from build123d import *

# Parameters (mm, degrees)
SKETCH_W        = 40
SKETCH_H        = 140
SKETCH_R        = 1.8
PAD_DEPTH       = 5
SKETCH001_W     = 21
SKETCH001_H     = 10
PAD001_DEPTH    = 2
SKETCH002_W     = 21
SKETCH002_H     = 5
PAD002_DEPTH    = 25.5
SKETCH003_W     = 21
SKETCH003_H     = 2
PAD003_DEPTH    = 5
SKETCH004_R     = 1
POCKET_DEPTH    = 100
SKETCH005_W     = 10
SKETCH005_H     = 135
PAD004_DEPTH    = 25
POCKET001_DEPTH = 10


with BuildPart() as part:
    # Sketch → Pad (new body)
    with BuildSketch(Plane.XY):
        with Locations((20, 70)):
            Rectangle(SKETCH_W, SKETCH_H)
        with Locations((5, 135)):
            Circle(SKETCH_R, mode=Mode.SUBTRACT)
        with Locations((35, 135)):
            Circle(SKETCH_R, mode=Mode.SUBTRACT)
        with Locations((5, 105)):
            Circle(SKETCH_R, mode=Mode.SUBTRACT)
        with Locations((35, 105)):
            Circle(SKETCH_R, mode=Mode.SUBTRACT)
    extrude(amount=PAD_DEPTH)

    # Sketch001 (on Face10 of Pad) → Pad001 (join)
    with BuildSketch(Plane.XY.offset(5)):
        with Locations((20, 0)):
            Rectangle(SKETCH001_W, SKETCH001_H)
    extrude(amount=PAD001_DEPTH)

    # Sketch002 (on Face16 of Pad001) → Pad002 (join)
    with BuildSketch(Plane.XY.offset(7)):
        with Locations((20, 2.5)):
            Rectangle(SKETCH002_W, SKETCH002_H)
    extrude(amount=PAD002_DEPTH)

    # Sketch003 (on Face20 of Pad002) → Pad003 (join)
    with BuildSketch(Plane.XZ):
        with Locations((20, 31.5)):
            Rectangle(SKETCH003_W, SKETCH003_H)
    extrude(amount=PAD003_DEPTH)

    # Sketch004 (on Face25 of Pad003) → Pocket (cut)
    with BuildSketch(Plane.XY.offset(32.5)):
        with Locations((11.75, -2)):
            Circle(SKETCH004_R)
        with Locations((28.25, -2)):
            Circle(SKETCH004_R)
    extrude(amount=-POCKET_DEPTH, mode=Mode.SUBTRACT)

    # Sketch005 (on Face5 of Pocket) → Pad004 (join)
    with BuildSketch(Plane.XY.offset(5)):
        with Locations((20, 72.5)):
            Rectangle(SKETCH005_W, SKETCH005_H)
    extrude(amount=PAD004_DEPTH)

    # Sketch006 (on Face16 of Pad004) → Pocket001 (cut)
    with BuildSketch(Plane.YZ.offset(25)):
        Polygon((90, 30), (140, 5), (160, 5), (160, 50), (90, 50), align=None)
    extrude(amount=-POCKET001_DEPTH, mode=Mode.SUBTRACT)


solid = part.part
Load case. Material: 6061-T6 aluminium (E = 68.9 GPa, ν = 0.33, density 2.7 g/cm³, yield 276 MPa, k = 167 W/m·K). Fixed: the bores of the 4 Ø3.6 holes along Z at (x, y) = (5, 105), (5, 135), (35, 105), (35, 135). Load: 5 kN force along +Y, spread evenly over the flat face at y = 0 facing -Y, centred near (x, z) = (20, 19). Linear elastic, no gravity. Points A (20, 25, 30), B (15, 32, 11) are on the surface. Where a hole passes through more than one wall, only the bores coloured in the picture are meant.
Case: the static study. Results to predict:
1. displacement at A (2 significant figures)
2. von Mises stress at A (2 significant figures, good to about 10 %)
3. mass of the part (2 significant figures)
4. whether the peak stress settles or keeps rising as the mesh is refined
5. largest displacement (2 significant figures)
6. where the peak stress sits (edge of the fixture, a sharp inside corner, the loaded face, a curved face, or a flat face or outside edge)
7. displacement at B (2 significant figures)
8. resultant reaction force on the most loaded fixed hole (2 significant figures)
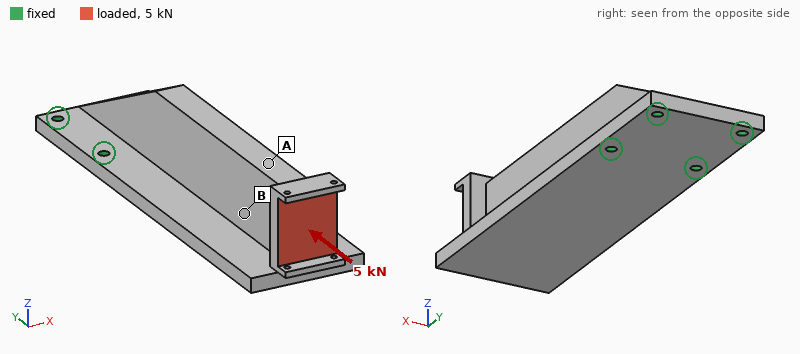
0.35 mm
30 MPa
160 g
keeps rising
0.49 mm
edge of the fixture
0.30 mm
1.8 kN
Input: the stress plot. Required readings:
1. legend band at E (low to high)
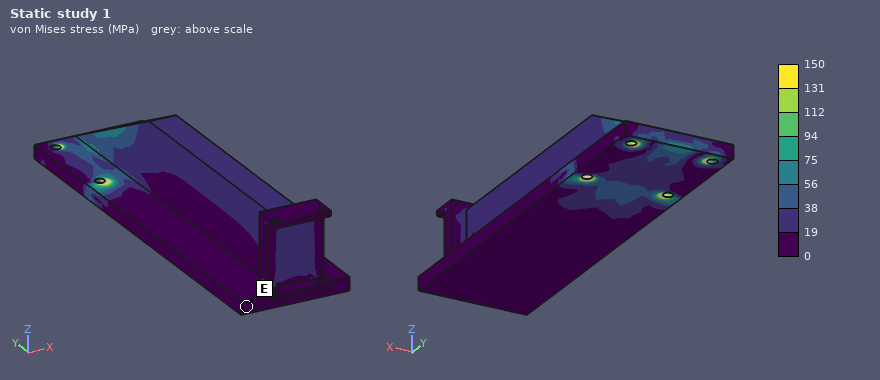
0 to 19 MPa
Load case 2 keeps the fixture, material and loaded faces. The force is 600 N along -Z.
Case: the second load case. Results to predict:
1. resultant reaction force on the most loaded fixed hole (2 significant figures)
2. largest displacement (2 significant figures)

1.5 kN
0.43 mm
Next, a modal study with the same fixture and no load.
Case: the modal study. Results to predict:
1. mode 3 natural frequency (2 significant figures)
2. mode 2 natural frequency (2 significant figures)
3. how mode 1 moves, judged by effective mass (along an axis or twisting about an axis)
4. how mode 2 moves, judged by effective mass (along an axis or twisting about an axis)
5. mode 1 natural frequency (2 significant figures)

2800 Hz
1500 Hz
along Z
along X
890 Hz
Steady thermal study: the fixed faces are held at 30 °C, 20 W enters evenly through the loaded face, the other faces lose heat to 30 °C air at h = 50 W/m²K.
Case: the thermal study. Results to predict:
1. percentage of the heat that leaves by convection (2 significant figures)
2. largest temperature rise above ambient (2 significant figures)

46 %
24 K
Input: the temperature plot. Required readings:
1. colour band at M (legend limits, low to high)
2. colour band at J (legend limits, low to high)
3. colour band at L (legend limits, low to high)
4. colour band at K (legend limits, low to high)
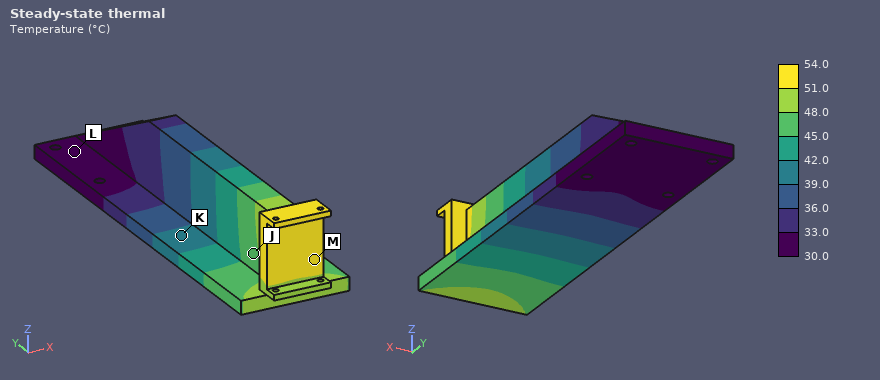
51.0 to 54.0 °C
45.0 to 48.0 °C
30.0 to 33.0 °C
39.0 to 42.0 °C
